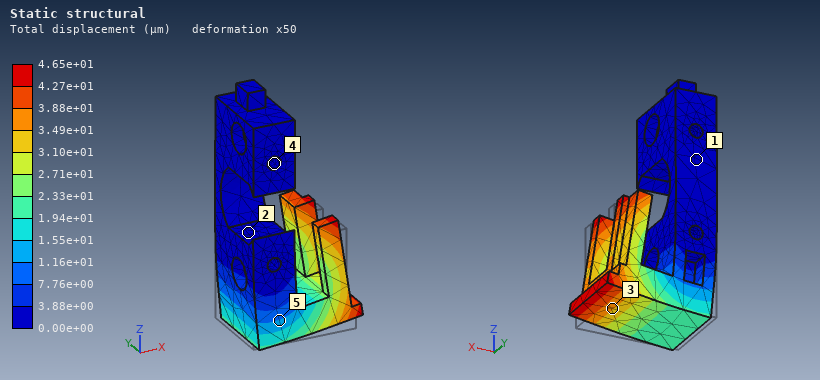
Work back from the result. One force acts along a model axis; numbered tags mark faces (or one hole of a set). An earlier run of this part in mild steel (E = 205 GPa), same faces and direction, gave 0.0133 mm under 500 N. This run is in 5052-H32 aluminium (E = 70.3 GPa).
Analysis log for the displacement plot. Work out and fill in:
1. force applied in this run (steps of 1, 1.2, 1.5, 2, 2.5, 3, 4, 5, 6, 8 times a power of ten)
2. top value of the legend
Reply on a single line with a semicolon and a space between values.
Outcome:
600 N; 4.65e+01 µm
